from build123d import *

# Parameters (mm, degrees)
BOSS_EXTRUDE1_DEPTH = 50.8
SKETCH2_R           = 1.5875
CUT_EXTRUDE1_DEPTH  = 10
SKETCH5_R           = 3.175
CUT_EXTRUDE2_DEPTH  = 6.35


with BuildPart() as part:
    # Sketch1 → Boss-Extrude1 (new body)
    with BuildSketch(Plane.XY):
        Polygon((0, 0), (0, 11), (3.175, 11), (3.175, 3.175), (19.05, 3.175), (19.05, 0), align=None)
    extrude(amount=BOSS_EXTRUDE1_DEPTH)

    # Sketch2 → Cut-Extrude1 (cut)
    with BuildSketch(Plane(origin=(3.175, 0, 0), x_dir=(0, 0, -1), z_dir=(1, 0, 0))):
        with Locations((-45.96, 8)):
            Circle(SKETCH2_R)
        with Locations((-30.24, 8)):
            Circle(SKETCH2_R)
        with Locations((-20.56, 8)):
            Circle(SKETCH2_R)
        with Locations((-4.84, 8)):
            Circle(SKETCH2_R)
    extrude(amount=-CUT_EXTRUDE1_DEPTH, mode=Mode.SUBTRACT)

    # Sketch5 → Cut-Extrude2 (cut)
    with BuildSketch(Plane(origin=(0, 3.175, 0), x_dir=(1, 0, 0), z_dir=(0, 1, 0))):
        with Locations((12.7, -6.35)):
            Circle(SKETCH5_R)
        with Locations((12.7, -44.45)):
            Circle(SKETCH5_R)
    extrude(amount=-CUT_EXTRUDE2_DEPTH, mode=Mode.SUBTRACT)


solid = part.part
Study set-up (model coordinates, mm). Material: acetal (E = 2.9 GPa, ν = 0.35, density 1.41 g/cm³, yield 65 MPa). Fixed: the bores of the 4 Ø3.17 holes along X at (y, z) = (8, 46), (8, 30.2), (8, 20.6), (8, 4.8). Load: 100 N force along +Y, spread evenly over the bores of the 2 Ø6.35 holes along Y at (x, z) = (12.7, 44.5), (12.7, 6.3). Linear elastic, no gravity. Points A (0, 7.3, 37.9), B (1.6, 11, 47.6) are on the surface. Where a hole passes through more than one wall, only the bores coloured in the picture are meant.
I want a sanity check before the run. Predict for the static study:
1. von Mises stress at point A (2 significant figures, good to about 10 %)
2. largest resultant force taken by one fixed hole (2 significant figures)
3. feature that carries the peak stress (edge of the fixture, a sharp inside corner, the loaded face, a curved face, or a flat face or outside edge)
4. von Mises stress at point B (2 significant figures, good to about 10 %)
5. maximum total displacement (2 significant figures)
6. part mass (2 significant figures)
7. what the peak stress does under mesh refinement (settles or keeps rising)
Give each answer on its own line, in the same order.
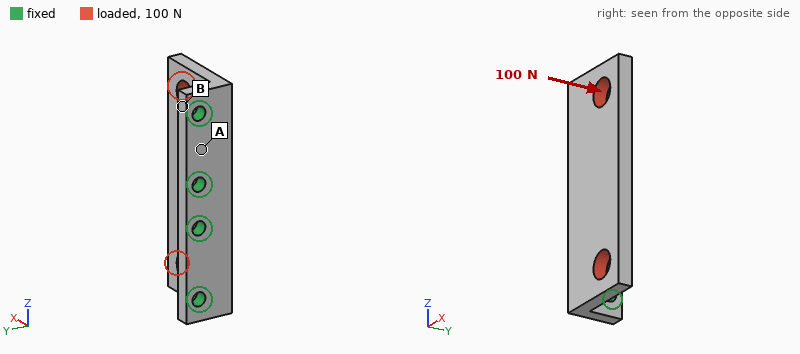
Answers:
4.5 MPa
41 N
edge of the fixture
2.5 MPa
0.56 mm
5.7 g
keeps rising
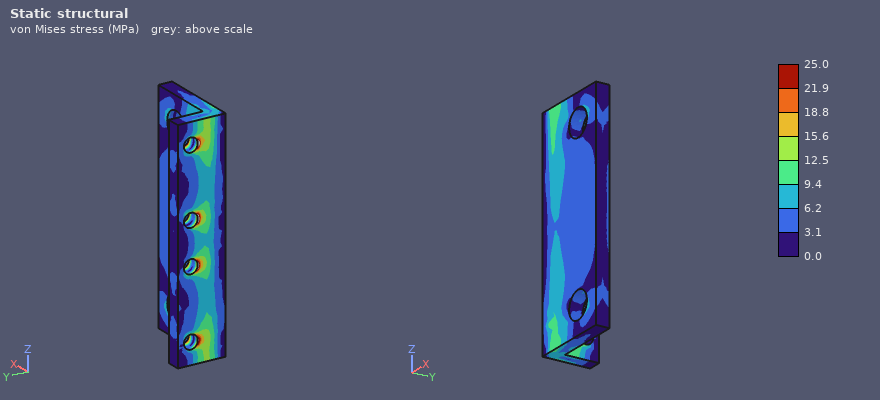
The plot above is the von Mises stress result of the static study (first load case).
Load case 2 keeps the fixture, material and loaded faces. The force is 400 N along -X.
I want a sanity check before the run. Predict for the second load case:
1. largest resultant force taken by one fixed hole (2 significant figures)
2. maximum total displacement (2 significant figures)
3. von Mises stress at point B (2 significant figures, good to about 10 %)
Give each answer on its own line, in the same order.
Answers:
120 N
0.40 mm
6.4 MPa
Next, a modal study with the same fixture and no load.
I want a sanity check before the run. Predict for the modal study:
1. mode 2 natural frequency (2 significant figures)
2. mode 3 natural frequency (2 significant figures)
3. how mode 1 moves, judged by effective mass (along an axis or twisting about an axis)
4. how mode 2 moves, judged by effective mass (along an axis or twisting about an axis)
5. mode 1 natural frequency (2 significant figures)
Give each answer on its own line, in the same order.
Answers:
2400 Hz
4200 Hz
along Y
twisting about X
1700 Hz
